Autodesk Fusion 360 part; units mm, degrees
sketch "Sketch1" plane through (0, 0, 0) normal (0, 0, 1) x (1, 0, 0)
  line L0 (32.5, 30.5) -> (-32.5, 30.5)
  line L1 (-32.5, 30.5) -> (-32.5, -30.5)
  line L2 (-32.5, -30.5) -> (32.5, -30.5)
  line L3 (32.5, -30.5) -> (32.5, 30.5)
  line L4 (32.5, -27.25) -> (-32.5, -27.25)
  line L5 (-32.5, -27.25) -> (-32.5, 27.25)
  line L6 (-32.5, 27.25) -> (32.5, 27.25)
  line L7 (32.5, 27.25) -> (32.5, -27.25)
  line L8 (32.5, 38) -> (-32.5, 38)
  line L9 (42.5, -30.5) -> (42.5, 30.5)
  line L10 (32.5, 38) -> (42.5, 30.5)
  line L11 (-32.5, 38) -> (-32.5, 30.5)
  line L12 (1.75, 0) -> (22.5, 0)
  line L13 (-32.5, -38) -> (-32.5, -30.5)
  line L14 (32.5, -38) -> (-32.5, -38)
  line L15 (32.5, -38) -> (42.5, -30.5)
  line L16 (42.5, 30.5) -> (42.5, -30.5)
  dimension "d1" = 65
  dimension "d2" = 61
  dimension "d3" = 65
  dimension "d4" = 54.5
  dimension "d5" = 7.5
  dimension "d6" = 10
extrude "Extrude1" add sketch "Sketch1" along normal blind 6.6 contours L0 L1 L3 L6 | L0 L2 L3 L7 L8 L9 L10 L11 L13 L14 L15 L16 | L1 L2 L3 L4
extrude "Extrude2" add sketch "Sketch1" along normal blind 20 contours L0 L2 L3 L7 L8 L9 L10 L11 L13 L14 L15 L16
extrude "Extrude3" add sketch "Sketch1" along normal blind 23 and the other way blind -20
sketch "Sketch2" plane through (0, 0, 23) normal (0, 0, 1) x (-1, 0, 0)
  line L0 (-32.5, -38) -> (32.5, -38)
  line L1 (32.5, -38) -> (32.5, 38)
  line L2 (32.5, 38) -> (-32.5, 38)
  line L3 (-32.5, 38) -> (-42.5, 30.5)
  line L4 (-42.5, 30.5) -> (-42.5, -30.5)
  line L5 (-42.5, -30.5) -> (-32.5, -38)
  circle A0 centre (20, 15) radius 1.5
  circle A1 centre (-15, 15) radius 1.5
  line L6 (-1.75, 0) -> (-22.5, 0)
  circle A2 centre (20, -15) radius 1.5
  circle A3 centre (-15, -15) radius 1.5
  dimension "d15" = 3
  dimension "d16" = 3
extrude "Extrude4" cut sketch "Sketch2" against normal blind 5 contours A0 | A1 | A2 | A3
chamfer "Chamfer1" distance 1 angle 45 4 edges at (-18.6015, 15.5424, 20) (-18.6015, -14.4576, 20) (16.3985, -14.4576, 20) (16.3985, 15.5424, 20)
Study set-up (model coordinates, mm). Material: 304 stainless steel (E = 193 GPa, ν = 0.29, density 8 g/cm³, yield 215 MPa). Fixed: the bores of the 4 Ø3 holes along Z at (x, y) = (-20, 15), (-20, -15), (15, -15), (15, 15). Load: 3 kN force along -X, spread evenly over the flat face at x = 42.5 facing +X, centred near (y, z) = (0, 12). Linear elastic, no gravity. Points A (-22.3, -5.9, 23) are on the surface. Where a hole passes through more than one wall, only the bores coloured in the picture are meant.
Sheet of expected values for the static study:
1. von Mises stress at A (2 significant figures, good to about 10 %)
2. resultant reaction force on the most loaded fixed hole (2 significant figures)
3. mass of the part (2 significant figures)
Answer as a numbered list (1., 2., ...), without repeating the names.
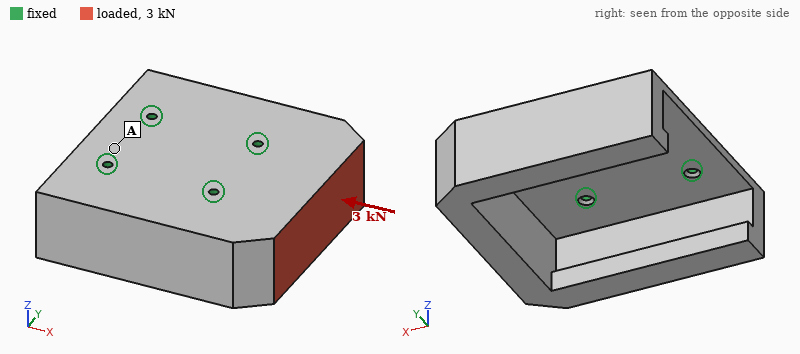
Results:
1. 14 MPa
2. 1.1 kN
3. 420 g
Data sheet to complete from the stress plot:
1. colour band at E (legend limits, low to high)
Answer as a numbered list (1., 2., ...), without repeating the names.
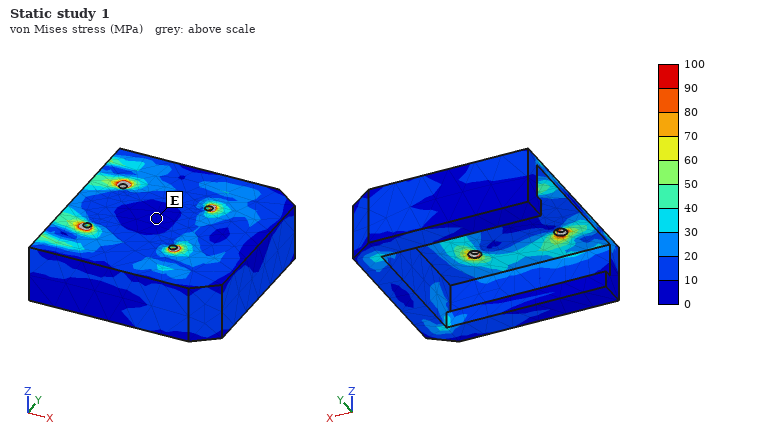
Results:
1. 0 to 10 MPa
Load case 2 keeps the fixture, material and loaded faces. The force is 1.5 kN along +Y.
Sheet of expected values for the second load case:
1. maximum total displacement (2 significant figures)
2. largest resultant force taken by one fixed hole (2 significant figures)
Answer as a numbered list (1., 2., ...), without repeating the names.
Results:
1. 37 µm
2. 1.2 kN
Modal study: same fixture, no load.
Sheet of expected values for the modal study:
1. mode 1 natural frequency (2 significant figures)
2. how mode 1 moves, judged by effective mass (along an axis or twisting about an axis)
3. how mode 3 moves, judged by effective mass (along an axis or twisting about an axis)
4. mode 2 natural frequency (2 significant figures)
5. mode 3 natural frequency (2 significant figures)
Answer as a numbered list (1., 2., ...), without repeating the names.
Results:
1. 1400 Hz
2. along Y
3. along Z
4. 1700 Hz
5. 2400 Hz
